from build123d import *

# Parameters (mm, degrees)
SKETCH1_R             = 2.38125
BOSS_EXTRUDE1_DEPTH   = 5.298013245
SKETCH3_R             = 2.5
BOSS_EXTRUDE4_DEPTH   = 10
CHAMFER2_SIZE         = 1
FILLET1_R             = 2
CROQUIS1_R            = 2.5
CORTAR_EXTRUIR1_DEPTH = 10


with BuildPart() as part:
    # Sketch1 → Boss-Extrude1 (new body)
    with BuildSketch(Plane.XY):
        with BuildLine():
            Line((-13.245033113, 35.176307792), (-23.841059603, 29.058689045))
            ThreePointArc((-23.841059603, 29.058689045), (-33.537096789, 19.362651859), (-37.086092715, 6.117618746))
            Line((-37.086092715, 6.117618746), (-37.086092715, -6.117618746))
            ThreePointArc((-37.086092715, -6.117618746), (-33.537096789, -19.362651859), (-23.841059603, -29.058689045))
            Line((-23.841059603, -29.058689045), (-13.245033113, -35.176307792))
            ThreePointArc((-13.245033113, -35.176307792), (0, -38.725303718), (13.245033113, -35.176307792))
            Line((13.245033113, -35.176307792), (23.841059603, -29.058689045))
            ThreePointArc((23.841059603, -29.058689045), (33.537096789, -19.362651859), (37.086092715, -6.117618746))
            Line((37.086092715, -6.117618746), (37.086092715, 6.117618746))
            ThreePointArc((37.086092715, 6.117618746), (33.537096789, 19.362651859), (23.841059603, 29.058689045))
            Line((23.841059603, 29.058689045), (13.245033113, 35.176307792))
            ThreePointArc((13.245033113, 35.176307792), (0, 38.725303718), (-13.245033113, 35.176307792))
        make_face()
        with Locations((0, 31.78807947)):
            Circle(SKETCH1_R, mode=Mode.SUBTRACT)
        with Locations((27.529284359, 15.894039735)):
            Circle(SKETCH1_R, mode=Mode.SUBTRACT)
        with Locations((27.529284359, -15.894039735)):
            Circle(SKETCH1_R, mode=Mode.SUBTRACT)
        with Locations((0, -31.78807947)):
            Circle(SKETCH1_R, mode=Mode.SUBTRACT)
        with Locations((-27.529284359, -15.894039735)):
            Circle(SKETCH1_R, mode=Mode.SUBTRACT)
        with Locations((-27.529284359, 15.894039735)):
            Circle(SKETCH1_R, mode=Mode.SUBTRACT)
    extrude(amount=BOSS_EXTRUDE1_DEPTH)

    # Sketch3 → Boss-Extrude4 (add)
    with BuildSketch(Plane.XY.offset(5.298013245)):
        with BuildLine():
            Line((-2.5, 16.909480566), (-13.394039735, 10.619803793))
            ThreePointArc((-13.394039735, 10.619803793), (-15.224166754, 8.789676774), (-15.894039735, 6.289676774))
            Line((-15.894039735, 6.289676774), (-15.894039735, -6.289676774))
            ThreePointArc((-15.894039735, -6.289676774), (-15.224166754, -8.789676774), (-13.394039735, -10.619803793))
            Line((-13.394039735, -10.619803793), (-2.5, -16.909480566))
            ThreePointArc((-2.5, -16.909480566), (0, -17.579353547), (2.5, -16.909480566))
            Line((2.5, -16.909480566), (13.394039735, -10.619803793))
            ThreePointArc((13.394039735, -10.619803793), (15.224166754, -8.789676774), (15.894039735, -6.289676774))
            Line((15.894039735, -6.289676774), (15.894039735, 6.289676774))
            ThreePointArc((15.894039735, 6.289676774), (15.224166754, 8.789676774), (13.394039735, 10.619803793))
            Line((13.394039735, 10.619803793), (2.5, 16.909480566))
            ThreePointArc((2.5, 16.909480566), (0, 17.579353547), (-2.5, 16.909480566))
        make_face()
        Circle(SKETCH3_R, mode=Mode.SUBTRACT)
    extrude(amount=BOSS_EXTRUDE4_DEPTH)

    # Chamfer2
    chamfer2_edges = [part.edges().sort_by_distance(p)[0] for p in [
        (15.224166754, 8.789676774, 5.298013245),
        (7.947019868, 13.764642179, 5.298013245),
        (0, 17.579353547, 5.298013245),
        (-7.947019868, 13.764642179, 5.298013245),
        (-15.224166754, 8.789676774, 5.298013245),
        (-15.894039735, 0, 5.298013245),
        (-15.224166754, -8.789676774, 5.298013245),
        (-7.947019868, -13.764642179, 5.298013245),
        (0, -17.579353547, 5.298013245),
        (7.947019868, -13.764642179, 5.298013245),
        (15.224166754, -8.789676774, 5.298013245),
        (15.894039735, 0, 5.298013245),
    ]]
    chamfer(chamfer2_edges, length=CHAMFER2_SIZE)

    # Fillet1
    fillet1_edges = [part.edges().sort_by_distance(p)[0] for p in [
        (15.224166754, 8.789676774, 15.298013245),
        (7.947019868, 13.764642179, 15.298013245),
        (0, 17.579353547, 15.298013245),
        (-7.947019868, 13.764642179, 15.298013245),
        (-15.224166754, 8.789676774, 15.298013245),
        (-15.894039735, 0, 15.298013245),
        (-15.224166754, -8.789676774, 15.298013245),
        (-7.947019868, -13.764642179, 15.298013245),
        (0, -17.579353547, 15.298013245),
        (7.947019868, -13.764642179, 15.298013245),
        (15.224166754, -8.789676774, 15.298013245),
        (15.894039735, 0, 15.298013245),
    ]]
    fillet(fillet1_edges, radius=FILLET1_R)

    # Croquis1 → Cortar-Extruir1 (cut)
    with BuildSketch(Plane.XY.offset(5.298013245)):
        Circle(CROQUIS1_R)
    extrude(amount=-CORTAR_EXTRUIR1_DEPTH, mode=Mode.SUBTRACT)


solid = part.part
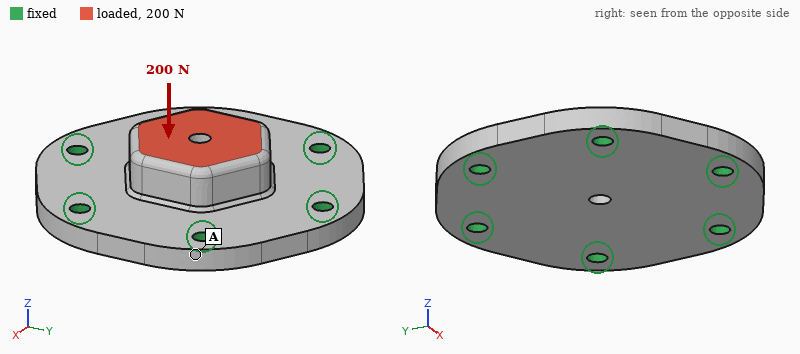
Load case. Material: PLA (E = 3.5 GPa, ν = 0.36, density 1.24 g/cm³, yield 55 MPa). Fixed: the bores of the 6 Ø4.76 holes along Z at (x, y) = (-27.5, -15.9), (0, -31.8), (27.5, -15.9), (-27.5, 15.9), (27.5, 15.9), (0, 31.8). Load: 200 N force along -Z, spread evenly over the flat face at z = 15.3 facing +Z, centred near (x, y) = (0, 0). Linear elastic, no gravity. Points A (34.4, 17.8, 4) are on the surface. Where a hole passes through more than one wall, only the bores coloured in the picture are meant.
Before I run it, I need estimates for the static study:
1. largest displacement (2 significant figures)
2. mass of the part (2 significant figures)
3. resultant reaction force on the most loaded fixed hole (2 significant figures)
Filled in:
22 µm
39 g
37 N
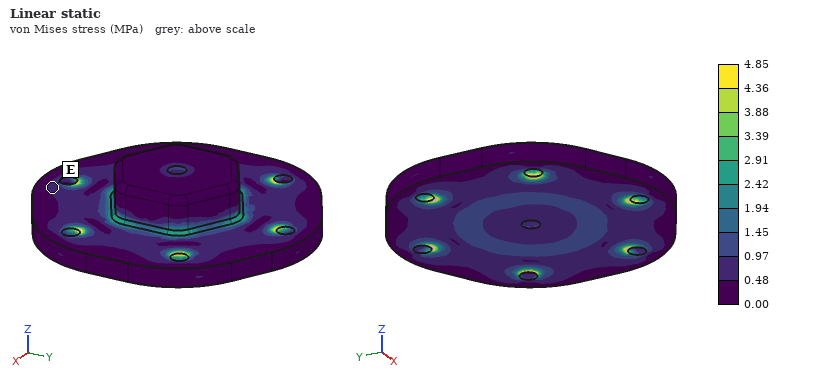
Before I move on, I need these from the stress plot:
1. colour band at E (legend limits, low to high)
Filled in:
0.48 to 0.97 MPa
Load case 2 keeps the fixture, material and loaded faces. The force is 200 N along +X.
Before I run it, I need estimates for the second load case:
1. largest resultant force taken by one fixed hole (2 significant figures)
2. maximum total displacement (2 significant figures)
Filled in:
53 N
18 µm
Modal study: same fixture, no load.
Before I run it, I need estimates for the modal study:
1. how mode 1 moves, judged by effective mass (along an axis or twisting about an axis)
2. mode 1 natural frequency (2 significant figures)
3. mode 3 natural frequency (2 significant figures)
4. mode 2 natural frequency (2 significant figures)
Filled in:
along Z
3500 Hz
5500 Hz
5500 Hz
